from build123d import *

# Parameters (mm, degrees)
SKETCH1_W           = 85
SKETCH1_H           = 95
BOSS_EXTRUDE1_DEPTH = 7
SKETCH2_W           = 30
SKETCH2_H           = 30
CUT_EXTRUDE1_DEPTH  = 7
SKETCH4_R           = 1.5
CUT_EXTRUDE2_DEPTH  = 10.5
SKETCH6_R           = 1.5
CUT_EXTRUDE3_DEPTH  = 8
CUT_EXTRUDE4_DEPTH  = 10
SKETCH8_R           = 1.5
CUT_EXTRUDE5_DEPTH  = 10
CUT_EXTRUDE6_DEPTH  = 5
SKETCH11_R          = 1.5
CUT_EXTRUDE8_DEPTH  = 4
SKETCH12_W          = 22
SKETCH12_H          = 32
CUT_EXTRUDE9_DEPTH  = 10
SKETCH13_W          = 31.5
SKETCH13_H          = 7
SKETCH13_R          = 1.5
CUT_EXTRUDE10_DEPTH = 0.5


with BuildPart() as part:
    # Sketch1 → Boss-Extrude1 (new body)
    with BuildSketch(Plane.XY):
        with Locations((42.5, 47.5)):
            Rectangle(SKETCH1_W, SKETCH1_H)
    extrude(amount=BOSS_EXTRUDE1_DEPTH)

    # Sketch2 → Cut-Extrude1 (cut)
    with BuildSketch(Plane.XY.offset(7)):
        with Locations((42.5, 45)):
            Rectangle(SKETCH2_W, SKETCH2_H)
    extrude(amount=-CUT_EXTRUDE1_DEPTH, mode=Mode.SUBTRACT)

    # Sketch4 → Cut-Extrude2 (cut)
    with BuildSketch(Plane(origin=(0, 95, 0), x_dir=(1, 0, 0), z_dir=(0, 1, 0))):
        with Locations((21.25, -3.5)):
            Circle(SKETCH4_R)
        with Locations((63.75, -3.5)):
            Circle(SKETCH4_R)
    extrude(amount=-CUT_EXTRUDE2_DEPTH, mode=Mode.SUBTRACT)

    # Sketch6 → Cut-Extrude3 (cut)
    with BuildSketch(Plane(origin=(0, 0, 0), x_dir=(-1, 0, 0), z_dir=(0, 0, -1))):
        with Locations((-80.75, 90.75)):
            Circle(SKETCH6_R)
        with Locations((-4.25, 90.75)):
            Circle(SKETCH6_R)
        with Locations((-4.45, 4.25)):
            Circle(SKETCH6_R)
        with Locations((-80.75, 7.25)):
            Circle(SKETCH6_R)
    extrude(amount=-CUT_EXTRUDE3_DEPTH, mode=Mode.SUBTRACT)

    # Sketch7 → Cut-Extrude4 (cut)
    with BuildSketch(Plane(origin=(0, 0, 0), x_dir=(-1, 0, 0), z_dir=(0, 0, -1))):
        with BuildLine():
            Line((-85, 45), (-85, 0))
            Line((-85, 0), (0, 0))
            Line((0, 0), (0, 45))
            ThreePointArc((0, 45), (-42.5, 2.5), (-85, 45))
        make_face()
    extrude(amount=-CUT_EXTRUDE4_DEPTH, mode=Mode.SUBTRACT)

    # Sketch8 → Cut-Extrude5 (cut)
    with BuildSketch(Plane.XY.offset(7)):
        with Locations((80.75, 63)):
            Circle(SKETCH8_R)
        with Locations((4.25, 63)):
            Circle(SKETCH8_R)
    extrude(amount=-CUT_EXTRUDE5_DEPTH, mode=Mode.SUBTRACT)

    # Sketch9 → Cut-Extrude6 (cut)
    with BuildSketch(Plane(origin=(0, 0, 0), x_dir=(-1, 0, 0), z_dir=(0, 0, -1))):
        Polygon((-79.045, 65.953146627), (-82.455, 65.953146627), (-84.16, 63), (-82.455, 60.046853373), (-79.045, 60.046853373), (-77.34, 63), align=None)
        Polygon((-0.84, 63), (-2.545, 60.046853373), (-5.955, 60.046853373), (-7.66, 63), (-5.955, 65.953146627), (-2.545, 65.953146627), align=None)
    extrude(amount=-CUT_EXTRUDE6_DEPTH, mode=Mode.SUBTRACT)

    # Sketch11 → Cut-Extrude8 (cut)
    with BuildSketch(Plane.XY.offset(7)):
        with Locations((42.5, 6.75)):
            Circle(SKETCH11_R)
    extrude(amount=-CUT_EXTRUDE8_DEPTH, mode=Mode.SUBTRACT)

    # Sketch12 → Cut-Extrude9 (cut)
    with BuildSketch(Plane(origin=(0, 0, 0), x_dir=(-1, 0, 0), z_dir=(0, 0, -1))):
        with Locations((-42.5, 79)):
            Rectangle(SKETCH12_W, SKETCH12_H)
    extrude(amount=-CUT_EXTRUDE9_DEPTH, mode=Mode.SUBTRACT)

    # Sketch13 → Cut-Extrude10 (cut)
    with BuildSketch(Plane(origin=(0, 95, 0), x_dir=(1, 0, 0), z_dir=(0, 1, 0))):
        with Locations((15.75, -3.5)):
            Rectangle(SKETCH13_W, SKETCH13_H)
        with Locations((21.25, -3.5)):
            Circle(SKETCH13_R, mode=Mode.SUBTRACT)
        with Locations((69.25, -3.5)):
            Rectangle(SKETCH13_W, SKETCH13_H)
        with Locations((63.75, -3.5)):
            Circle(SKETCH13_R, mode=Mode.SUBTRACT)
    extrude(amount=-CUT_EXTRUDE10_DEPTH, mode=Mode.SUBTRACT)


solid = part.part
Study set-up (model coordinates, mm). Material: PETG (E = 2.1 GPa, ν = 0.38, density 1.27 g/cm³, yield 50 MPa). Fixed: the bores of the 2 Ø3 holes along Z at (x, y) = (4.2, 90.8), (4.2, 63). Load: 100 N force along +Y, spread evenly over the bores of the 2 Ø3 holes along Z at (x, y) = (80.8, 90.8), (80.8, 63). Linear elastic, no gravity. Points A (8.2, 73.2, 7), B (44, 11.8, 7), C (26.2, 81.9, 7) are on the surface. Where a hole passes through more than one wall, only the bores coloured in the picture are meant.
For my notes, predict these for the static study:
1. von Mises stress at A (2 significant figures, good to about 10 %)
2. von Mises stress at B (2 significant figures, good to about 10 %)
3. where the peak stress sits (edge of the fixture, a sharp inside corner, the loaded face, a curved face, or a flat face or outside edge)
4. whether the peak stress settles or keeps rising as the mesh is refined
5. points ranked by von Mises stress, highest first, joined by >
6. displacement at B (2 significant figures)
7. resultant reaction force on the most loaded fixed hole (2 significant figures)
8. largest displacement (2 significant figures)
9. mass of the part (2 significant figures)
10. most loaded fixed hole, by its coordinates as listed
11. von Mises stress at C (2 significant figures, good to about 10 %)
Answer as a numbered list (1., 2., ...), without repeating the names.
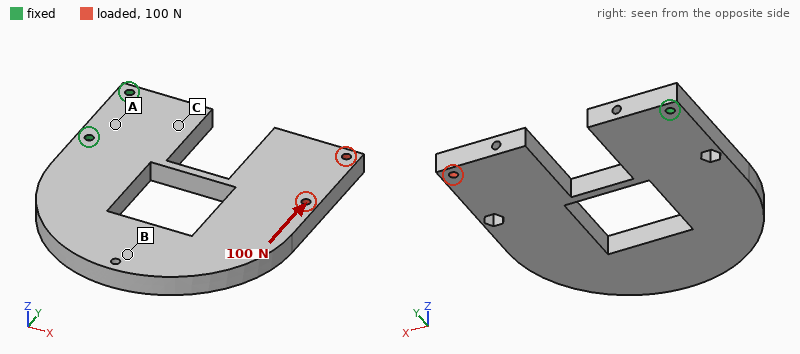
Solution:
1. 4.6 MPa
2. 1.2 MPa
3. edge of the fixture
4. keeps rising
5. A > C > B
6. 1.1 mm
7. 310 N
8. 1.5 mm
9. 48 g
10. (4.2, 90.8)
11. 2.6 MPa
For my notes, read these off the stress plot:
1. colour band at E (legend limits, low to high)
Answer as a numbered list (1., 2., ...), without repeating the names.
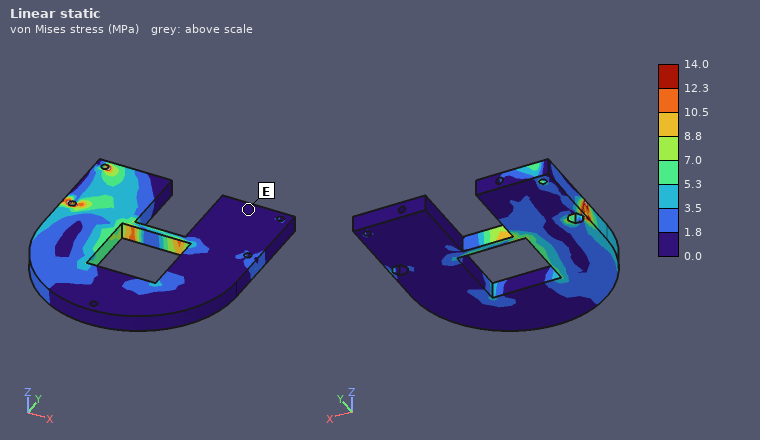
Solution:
1. 0.0 to 1.8 MPa
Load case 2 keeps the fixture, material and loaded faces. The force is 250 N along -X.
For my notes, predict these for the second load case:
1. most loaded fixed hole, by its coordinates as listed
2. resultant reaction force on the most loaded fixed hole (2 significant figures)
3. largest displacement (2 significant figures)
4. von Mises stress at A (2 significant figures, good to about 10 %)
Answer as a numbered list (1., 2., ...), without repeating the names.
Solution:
1. (4.2, 90.8)
2. 220 N
3. 1.4 mm
4. 1.8 MPa
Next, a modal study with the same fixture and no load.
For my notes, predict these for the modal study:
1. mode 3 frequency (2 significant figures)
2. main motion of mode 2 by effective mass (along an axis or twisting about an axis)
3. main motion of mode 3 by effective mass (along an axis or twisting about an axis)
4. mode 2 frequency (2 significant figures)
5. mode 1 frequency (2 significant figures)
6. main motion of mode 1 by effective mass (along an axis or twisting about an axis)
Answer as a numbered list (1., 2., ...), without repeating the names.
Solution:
1. 330 Hz
2. twisting about X
3. along Y
4. 180 Hz
5. 97 Hz
6. along Z
